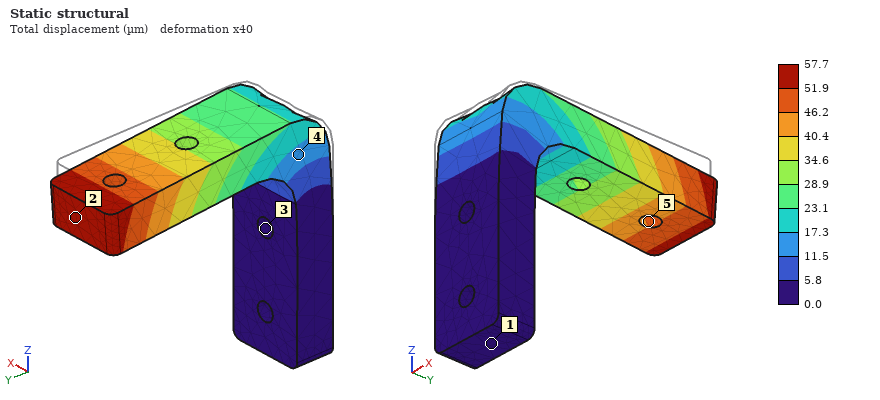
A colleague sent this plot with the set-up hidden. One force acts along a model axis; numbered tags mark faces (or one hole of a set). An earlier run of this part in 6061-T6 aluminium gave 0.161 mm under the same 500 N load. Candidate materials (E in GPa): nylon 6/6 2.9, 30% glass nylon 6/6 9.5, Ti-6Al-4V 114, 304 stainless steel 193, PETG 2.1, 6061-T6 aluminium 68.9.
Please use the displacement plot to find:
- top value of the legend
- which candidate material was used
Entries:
57.7 µm
304 stainless steel
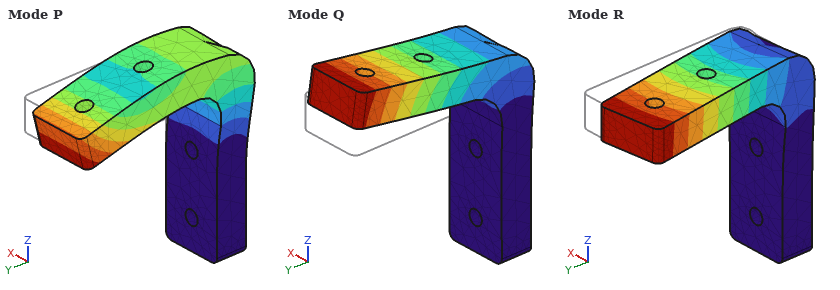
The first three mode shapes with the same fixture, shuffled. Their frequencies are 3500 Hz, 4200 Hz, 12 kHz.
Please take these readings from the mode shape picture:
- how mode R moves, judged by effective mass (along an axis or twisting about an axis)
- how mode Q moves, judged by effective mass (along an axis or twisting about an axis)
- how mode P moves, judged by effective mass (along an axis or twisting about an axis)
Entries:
along X
along Z
along Y
